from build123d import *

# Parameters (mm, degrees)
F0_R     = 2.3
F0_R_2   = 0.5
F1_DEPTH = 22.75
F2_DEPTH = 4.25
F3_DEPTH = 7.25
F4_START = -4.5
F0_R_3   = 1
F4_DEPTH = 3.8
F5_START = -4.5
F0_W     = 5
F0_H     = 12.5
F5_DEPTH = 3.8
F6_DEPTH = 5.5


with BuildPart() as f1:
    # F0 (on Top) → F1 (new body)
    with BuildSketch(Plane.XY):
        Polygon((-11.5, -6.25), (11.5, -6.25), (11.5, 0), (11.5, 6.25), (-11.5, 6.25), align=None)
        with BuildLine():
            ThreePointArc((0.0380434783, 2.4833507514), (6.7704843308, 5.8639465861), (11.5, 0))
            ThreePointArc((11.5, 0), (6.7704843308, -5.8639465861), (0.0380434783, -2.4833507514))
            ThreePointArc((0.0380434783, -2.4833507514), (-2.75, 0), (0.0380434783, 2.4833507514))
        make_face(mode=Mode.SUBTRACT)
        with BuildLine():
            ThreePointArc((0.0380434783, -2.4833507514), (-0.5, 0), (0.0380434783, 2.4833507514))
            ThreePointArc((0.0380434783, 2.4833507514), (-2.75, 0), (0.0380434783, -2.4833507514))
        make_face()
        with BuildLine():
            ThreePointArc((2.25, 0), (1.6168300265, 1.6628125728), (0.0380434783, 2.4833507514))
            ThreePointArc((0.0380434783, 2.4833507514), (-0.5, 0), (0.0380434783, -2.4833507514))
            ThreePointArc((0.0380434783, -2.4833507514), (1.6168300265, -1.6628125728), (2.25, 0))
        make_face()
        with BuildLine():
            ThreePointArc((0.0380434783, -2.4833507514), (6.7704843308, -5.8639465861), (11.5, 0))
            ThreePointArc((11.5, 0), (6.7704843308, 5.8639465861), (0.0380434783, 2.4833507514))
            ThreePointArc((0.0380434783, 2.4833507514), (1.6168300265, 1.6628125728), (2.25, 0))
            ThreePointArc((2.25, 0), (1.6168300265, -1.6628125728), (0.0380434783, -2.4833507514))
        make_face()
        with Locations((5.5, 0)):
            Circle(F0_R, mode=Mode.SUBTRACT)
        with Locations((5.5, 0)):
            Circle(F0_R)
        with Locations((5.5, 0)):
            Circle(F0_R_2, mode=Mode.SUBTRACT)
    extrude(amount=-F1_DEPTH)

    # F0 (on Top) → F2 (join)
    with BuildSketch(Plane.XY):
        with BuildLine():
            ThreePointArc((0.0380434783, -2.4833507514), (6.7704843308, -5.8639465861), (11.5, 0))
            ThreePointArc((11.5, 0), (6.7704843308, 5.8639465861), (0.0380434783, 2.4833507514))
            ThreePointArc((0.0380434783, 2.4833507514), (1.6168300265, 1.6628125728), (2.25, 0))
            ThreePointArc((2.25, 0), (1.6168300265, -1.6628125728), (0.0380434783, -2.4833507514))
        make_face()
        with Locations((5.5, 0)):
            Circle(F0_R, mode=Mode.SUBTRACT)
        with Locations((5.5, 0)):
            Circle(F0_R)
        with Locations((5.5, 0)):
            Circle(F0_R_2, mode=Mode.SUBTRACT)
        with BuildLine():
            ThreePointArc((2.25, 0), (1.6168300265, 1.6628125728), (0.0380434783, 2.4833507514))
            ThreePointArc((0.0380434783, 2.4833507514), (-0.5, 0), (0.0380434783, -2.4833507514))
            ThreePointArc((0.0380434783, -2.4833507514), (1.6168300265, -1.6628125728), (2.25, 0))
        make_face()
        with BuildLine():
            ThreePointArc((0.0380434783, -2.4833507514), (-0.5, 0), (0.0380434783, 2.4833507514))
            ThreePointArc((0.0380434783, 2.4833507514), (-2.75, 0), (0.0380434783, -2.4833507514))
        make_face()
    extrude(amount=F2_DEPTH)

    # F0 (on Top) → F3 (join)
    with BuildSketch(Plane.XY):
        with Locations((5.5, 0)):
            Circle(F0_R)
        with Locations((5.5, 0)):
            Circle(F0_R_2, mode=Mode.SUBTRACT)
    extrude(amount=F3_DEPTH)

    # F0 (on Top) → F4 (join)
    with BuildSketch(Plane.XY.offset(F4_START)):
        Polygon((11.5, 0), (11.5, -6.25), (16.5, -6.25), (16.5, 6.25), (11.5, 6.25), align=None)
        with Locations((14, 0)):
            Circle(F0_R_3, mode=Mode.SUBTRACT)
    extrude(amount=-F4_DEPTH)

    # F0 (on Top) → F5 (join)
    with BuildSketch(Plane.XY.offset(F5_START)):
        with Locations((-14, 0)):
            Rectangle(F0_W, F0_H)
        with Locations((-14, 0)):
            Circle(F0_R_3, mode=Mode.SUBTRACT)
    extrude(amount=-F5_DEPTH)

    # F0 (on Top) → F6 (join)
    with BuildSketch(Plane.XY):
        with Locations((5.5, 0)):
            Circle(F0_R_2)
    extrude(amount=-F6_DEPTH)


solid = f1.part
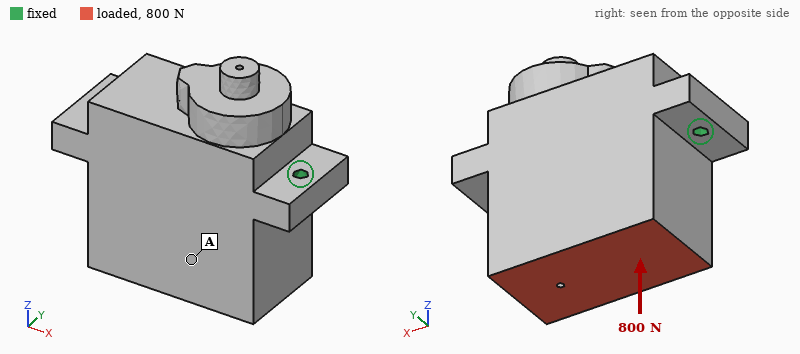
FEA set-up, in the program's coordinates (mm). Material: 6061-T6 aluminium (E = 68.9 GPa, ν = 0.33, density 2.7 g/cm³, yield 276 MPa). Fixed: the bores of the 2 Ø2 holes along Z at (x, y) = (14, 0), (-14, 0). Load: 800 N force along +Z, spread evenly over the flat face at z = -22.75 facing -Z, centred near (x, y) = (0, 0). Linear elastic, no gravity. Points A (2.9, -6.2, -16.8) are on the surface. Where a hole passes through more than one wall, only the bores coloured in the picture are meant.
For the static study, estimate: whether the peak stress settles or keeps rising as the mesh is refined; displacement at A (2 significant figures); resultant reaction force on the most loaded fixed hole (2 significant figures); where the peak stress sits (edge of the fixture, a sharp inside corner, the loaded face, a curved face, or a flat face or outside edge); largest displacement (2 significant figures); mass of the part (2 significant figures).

keeps rising
3.2 µm
400 N
edge of the fixture
3.4 µm
20 g
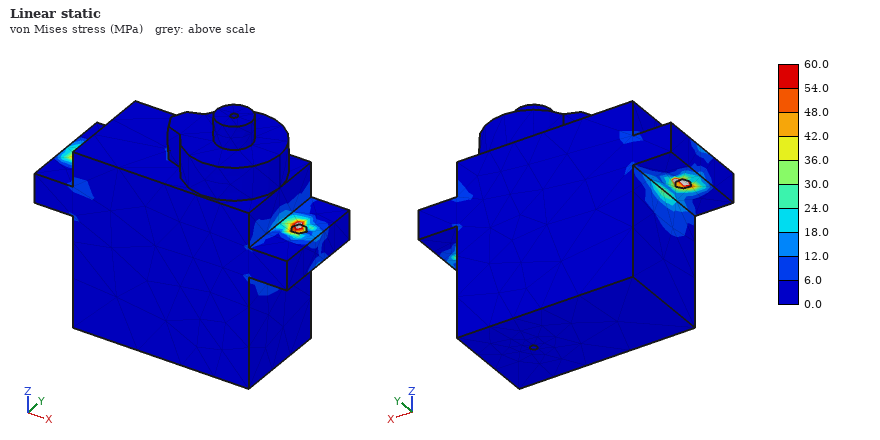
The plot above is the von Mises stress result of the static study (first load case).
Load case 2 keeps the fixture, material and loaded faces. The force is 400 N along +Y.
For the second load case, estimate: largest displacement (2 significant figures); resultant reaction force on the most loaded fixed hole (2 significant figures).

52 µm
200 N
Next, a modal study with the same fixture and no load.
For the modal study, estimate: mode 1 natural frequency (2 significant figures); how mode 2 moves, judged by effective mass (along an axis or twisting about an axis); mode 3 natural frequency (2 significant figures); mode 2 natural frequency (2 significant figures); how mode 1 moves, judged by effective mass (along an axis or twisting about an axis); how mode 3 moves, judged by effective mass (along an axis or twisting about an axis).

6100 Hz
along Z
20 kHz
19 kHz
along Y
along Y
